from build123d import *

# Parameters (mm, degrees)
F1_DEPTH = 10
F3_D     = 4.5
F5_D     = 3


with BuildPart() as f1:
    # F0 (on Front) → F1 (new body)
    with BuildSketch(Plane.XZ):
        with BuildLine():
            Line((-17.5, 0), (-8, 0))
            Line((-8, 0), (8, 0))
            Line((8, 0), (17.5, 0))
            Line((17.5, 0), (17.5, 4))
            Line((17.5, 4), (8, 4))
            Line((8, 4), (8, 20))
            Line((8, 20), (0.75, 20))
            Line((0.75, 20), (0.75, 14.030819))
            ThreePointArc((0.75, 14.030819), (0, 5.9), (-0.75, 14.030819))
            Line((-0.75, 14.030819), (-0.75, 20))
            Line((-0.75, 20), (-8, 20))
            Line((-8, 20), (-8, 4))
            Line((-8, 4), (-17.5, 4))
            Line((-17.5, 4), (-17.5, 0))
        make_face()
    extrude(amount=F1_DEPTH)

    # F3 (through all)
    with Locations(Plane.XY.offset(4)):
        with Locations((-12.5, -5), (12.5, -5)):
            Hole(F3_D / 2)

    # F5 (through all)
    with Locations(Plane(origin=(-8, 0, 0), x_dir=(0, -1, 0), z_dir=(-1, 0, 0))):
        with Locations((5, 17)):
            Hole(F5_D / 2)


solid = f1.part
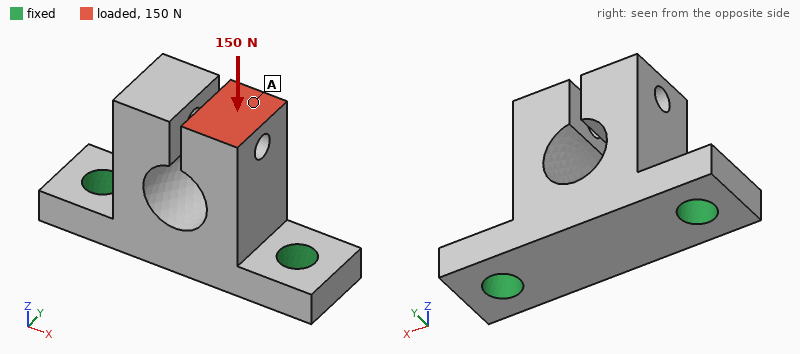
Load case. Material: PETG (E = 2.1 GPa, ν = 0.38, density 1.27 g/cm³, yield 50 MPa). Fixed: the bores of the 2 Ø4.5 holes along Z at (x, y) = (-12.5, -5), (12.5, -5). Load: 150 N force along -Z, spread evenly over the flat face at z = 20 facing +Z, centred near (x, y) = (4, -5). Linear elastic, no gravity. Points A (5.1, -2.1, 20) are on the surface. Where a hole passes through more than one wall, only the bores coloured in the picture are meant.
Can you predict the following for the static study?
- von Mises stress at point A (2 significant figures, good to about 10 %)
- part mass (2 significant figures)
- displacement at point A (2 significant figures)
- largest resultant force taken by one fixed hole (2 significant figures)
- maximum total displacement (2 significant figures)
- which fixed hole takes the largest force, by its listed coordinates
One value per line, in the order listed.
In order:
2.8 MPa
4.0 g
0.18 mm
120 N
0.22 mm
(12.5, -5)
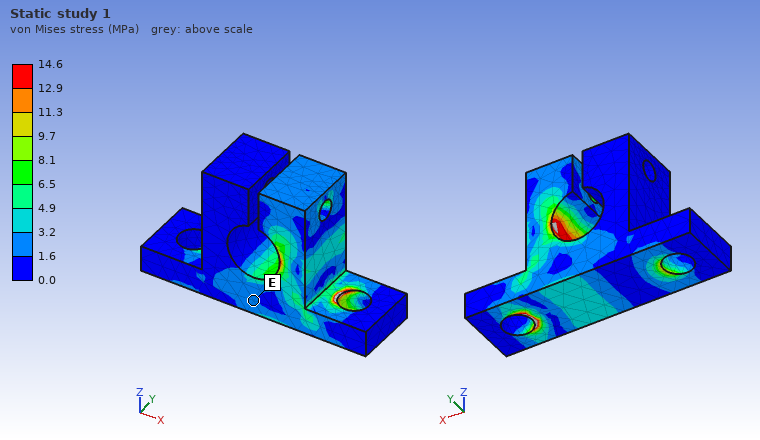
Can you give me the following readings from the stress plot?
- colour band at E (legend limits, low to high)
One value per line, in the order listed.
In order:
1.6 to 3.2 MPa
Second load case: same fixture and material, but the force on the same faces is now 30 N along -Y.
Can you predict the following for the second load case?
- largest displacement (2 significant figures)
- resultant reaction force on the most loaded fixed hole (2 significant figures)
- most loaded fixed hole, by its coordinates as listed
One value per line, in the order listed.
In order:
0.25 mm
21 N
(12.5, -5)
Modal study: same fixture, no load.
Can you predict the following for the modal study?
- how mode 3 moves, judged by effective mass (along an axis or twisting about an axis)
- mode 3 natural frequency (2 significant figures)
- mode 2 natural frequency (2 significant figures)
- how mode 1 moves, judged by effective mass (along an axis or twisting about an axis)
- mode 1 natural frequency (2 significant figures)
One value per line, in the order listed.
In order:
along X
2900 Hz
2700 Hz
along Y
2200 Hz
